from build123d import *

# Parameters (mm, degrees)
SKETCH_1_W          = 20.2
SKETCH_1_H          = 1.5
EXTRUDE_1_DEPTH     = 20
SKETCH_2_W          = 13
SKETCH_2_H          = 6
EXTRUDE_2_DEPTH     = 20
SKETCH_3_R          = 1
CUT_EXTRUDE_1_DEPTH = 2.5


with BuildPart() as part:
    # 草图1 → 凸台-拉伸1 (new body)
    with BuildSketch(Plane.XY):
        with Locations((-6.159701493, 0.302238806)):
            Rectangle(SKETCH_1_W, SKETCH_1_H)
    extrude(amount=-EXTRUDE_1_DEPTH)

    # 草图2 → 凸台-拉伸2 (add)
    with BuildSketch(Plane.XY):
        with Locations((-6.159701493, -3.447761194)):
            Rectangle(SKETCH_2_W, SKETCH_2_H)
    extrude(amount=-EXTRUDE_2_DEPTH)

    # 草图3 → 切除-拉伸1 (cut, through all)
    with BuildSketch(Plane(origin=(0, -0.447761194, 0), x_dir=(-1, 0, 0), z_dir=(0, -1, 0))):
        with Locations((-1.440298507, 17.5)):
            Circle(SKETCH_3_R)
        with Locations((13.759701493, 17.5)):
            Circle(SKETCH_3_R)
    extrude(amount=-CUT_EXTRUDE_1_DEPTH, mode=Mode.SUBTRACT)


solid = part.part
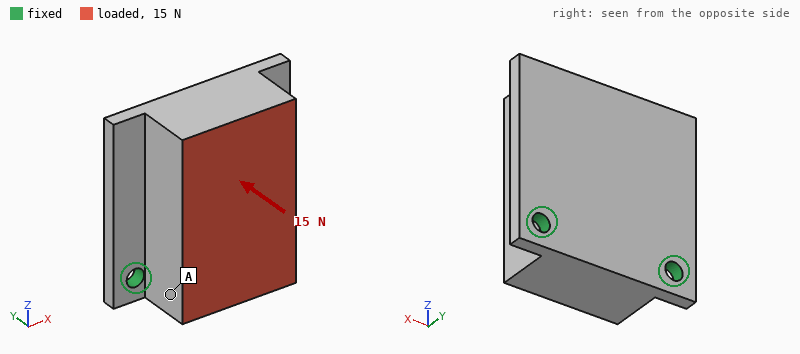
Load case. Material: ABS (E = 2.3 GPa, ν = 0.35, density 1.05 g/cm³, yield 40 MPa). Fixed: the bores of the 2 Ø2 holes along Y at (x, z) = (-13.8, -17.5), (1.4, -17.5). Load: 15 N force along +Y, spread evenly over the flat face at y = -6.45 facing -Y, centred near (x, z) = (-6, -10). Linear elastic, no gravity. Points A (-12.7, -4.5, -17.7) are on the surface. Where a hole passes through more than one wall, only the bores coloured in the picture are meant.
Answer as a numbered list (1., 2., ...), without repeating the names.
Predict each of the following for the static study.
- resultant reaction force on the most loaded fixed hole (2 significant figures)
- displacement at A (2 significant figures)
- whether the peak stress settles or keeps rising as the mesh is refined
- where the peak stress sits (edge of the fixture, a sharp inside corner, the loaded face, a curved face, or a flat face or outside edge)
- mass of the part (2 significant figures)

1. 8.0 N
2. 0.043 mm
3. keeps rising
4. edge of the fixture
5. 2.3 g
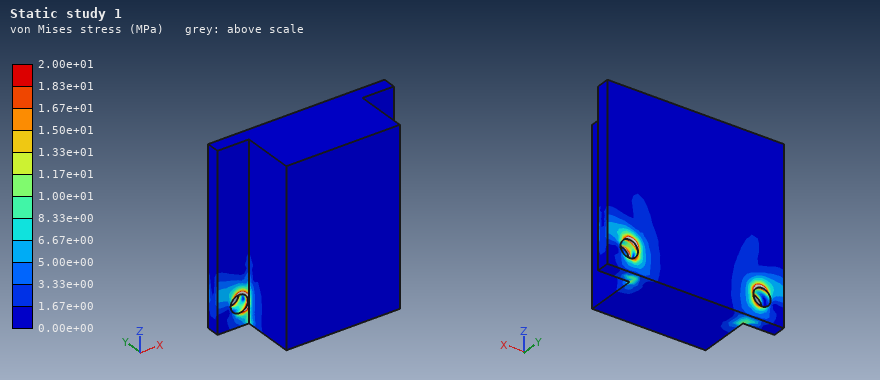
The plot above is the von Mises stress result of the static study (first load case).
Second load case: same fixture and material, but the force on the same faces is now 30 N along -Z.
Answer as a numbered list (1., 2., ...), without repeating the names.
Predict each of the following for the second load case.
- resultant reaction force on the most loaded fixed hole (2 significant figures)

1. 15 N
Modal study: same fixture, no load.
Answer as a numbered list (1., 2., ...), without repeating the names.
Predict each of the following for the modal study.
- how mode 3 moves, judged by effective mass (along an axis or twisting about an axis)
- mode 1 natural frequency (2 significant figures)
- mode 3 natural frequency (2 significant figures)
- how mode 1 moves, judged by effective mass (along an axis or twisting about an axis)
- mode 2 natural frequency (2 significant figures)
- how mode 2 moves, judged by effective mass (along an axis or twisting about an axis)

1. twisting about Z
2. 1100 Hz
3. 7300 Hz
4. along Y
5. 6000 Hz
6. along X
